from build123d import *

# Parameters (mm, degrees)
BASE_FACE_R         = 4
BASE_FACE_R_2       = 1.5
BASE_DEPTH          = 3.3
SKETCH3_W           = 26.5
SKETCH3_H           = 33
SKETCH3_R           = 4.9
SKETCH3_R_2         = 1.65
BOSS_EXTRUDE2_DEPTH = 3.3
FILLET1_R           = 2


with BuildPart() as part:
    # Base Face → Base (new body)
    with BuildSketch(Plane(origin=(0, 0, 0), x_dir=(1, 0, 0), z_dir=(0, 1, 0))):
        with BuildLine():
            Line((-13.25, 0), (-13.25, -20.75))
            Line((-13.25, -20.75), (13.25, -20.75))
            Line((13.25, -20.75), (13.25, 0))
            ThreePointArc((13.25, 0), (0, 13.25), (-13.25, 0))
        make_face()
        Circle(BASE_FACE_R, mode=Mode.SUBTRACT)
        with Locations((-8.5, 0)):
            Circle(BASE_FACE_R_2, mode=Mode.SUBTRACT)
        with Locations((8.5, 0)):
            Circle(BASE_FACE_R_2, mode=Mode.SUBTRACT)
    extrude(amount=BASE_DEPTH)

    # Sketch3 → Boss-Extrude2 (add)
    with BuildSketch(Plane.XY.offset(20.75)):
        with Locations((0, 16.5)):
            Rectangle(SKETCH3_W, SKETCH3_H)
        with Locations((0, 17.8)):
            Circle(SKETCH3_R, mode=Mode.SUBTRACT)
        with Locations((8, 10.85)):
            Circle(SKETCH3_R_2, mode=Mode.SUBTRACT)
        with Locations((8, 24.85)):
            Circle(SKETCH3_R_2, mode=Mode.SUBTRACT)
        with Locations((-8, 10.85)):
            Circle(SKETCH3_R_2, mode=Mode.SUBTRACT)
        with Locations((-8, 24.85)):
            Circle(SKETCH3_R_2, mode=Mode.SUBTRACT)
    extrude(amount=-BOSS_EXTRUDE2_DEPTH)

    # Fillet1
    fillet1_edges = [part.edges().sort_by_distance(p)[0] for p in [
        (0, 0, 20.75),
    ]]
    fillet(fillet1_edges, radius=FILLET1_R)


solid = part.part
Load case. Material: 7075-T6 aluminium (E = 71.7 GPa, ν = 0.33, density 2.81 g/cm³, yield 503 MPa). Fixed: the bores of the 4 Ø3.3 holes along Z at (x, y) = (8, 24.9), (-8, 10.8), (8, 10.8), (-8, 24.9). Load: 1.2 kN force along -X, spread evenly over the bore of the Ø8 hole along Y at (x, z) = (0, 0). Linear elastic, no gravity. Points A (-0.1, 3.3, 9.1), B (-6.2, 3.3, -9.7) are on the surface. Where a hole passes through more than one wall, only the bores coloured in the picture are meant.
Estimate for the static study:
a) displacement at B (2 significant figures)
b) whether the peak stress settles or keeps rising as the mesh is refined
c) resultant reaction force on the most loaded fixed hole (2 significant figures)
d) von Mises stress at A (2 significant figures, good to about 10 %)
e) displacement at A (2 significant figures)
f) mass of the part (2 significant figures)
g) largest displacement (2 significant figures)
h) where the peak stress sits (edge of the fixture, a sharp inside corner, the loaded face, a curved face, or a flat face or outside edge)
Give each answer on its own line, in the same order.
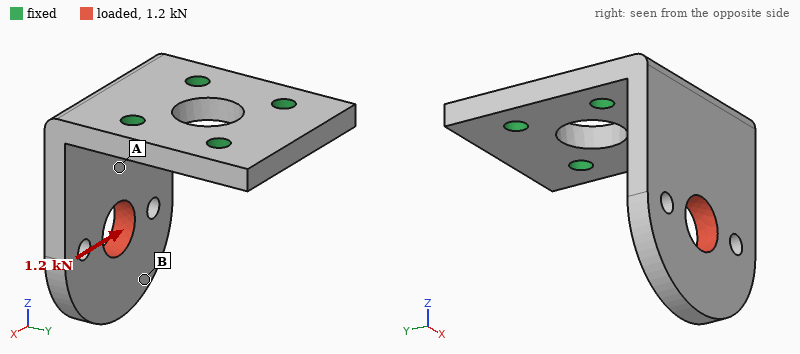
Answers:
0.24 mm
keeps rising
1.5 kN
75 MPa
0.085 mm
13 g
0.26 mm
edge of the fixture
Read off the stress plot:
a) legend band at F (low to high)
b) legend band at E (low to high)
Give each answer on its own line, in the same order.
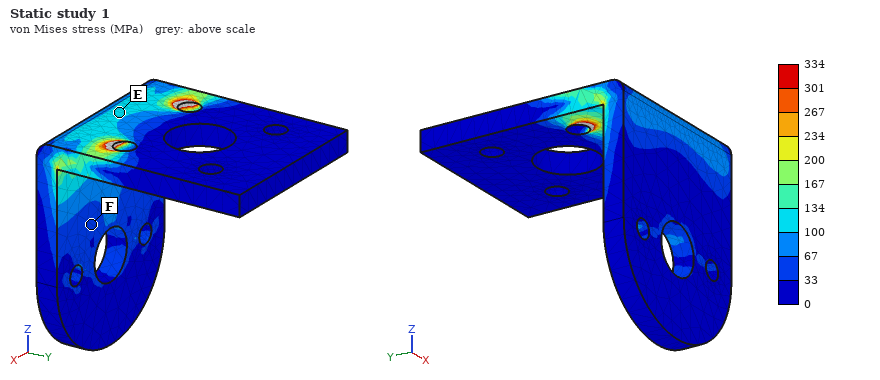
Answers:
33 to 67 MPa
100 to 134 MPa
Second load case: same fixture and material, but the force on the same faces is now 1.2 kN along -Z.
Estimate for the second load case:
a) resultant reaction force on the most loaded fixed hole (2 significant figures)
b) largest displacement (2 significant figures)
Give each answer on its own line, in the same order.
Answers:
650 N
0.28 mm
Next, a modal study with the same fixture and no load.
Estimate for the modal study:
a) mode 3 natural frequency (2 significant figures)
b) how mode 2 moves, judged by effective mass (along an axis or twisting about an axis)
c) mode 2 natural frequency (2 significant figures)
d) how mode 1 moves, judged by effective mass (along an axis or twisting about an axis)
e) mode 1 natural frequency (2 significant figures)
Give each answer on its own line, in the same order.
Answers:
8400 Hz
along X
5400 Hz
along Y
2200 Hz
